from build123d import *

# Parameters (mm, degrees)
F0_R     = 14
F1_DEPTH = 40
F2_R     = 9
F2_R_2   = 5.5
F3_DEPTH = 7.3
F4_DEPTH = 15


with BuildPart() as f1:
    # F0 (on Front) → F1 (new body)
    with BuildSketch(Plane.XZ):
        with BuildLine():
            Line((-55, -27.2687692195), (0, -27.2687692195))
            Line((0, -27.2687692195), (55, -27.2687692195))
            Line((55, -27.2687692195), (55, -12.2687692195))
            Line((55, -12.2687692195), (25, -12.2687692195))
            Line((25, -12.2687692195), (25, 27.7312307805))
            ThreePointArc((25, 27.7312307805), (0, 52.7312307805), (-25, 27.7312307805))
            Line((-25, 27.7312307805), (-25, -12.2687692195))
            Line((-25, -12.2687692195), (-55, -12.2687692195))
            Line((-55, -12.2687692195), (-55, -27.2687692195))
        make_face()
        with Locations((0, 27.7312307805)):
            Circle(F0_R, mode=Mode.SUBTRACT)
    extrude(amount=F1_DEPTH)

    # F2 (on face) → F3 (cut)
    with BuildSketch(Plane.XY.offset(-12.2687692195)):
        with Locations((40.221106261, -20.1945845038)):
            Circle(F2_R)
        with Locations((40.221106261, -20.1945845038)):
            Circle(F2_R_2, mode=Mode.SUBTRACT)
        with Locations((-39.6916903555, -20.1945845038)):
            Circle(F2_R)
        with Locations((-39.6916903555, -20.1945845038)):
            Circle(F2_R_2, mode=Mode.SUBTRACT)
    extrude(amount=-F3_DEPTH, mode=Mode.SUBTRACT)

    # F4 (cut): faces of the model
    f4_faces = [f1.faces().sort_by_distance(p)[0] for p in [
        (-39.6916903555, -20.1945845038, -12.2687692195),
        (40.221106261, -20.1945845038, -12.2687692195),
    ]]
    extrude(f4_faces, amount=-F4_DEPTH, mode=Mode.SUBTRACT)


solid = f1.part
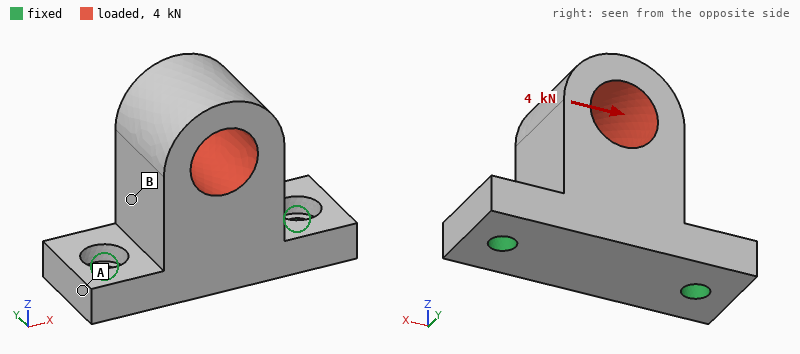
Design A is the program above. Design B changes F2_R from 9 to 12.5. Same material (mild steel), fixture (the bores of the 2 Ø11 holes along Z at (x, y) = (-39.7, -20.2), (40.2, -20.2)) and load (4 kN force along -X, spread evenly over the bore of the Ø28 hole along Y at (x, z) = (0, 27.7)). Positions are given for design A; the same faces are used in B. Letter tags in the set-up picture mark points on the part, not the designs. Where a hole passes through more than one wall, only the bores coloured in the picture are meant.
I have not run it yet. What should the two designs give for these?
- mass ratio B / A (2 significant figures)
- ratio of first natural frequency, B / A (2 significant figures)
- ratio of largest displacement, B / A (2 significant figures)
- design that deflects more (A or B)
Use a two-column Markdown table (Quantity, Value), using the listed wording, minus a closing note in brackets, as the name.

| Quantity | Value |
|---|---|
| mass ratio B / A | 0.98 |
| ratio of first natural frequency, B / A | 0.94 |
| ratio of largest displacement, B / A | 1.1 |
| design that deflects more | B |
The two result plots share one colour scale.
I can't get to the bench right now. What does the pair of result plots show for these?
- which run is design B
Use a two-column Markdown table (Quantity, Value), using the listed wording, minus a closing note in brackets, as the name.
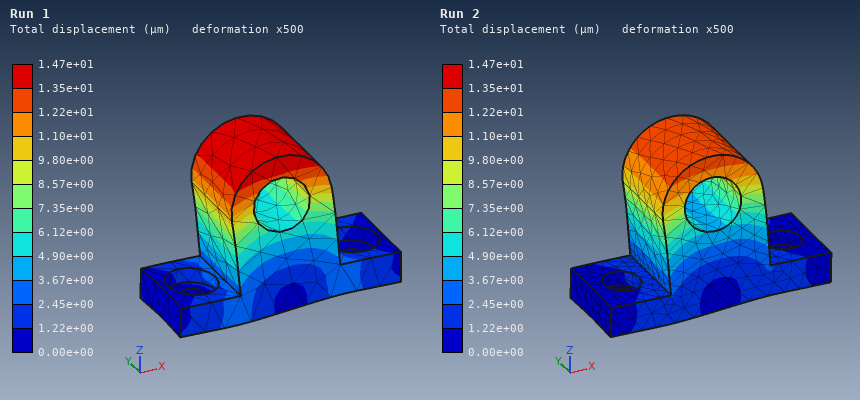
| Quantity | Value |
|---|---|
| which run is design B | Run 1 |
